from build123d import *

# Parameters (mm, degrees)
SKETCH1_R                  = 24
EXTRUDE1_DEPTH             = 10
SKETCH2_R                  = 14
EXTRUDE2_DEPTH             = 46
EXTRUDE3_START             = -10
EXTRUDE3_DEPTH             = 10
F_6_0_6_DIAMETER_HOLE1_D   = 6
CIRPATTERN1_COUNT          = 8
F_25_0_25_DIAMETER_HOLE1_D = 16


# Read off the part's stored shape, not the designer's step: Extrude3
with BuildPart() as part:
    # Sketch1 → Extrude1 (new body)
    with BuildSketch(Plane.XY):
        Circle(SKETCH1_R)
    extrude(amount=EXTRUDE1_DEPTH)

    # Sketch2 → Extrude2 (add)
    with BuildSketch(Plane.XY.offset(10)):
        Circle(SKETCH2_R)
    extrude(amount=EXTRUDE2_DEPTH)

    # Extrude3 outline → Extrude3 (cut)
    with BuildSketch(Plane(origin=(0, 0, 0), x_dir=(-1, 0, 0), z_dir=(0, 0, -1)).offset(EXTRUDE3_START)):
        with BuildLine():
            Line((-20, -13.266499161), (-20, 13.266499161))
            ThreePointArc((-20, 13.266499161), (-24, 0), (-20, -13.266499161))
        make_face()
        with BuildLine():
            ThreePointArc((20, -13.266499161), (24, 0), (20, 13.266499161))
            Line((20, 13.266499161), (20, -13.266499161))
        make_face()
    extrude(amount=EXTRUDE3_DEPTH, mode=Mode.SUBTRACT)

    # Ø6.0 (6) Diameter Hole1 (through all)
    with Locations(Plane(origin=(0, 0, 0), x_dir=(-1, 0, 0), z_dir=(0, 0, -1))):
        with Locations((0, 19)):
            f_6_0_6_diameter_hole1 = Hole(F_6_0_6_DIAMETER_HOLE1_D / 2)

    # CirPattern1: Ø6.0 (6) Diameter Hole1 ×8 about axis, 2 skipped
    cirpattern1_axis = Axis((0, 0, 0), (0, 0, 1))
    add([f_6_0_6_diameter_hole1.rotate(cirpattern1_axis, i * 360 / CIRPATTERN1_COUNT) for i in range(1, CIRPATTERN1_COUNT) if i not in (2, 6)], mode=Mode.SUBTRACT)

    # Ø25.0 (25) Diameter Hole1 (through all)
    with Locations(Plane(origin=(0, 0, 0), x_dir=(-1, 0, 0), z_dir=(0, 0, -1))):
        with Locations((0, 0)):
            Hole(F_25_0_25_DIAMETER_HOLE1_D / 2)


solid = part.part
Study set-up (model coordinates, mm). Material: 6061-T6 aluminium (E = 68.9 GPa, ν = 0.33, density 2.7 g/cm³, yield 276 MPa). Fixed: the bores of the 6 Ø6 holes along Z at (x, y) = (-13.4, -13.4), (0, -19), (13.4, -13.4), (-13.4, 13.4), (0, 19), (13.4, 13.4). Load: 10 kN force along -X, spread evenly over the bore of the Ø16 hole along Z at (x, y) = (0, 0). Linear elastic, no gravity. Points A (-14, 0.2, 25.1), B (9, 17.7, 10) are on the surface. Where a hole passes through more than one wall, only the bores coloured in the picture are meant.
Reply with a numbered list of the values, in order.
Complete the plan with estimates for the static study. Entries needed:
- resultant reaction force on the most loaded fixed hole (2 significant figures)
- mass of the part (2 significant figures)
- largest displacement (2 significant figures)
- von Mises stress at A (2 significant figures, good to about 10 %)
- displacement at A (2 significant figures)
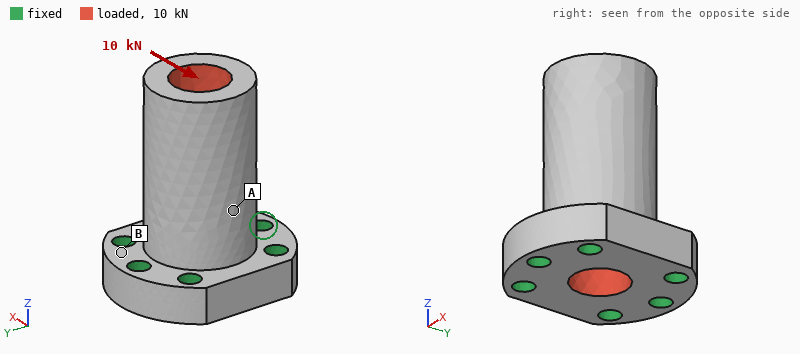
1. 4.9 kN
2. 86 g
3. 0.13 mm
4. 41 MPa
5. 0.053 mm
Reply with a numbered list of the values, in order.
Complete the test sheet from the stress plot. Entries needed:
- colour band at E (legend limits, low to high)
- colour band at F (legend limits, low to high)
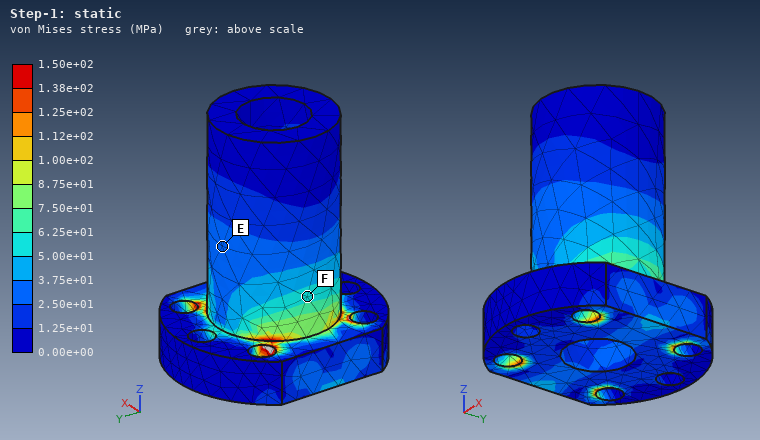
1. 2.50e+01 to 3.75e+01 MPa
2. 5.00e+01 to 6.25e+01 MPa
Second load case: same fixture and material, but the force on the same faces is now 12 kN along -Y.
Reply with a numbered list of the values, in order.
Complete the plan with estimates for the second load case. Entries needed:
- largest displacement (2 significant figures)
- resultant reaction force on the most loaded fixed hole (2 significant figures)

1. 0.14 mm
2. 5.0 kN
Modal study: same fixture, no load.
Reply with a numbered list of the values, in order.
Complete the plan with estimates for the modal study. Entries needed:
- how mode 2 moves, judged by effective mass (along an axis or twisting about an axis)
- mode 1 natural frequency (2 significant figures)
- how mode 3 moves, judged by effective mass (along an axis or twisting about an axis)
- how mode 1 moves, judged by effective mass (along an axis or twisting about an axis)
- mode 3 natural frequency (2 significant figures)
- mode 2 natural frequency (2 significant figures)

1. along Y
2. 6600 Hz
3. twisting about Z
4. along X
5. 16 kHz
6. 7100 Hz
